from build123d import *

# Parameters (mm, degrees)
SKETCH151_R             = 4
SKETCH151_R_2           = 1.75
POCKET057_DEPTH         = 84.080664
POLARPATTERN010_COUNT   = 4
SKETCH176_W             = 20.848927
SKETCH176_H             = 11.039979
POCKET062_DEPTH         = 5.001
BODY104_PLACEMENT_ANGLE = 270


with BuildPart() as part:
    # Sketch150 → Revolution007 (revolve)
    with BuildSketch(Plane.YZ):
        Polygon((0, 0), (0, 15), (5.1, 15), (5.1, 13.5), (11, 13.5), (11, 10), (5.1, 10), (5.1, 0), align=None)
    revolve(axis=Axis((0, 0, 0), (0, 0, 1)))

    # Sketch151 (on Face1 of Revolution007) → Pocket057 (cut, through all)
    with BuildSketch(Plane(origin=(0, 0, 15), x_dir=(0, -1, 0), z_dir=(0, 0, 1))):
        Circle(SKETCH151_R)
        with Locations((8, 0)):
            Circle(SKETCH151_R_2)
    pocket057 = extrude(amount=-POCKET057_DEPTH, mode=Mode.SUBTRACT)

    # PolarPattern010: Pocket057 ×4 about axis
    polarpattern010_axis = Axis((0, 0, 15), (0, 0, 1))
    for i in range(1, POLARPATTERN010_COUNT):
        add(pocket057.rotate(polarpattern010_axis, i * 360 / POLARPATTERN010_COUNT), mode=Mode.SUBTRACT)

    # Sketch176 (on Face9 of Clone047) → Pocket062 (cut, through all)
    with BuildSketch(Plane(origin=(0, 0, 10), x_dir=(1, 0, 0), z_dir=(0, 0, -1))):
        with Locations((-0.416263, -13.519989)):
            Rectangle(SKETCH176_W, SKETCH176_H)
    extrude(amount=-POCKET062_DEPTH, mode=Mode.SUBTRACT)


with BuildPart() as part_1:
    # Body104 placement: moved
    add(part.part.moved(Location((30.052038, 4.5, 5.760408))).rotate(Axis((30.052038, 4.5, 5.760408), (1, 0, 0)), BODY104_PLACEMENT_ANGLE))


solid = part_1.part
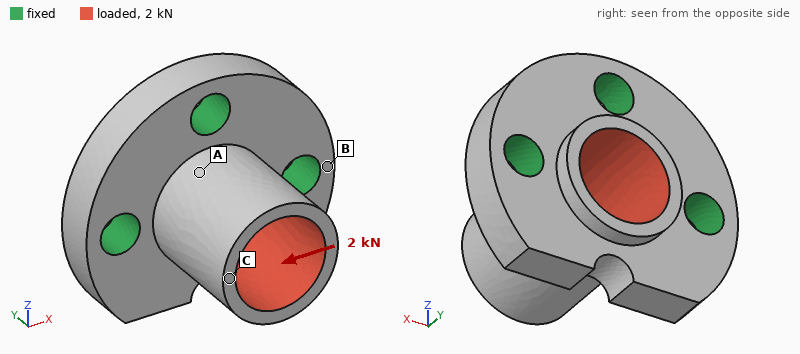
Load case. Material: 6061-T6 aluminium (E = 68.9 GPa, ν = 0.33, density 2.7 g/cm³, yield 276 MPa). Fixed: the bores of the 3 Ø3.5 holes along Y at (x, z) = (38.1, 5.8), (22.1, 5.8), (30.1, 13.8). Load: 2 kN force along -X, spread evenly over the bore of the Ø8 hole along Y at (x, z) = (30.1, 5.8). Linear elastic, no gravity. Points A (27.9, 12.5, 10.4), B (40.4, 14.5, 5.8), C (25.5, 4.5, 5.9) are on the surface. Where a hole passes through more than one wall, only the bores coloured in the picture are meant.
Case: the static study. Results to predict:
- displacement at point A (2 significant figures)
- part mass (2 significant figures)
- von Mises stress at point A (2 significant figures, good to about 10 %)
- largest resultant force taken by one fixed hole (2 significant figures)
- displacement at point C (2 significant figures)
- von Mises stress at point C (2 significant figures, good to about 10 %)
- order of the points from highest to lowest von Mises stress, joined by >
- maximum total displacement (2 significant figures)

10 µm
3.5 g
80 MPa
1.0 kN
36 µm
28 MPa
A > C > B
36 µm
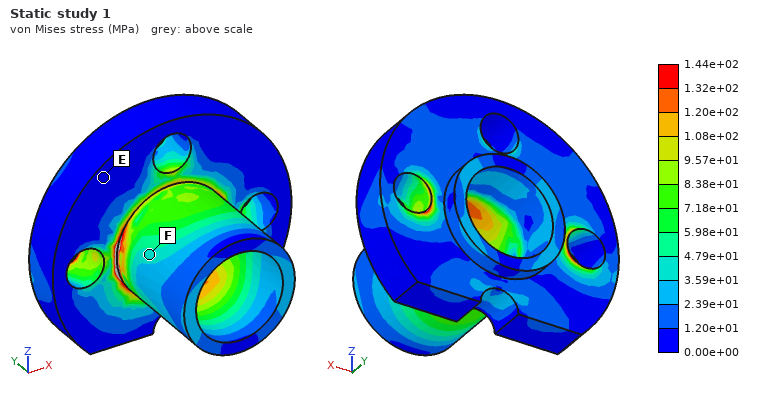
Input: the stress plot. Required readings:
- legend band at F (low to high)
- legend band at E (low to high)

3.59e+01 to 4.79e+01 MPa
0.00e+00 to 1.20e+01 MPa
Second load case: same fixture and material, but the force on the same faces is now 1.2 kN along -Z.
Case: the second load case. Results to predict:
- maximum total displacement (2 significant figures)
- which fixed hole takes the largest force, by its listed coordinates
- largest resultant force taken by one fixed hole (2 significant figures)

36 µm
(30.1, 13.8)
590 N
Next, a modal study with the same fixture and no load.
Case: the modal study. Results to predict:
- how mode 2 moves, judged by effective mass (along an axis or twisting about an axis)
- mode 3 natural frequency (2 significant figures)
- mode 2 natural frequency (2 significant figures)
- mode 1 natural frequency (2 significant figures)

along X
41 kHz
39 kHz
28 kHz
